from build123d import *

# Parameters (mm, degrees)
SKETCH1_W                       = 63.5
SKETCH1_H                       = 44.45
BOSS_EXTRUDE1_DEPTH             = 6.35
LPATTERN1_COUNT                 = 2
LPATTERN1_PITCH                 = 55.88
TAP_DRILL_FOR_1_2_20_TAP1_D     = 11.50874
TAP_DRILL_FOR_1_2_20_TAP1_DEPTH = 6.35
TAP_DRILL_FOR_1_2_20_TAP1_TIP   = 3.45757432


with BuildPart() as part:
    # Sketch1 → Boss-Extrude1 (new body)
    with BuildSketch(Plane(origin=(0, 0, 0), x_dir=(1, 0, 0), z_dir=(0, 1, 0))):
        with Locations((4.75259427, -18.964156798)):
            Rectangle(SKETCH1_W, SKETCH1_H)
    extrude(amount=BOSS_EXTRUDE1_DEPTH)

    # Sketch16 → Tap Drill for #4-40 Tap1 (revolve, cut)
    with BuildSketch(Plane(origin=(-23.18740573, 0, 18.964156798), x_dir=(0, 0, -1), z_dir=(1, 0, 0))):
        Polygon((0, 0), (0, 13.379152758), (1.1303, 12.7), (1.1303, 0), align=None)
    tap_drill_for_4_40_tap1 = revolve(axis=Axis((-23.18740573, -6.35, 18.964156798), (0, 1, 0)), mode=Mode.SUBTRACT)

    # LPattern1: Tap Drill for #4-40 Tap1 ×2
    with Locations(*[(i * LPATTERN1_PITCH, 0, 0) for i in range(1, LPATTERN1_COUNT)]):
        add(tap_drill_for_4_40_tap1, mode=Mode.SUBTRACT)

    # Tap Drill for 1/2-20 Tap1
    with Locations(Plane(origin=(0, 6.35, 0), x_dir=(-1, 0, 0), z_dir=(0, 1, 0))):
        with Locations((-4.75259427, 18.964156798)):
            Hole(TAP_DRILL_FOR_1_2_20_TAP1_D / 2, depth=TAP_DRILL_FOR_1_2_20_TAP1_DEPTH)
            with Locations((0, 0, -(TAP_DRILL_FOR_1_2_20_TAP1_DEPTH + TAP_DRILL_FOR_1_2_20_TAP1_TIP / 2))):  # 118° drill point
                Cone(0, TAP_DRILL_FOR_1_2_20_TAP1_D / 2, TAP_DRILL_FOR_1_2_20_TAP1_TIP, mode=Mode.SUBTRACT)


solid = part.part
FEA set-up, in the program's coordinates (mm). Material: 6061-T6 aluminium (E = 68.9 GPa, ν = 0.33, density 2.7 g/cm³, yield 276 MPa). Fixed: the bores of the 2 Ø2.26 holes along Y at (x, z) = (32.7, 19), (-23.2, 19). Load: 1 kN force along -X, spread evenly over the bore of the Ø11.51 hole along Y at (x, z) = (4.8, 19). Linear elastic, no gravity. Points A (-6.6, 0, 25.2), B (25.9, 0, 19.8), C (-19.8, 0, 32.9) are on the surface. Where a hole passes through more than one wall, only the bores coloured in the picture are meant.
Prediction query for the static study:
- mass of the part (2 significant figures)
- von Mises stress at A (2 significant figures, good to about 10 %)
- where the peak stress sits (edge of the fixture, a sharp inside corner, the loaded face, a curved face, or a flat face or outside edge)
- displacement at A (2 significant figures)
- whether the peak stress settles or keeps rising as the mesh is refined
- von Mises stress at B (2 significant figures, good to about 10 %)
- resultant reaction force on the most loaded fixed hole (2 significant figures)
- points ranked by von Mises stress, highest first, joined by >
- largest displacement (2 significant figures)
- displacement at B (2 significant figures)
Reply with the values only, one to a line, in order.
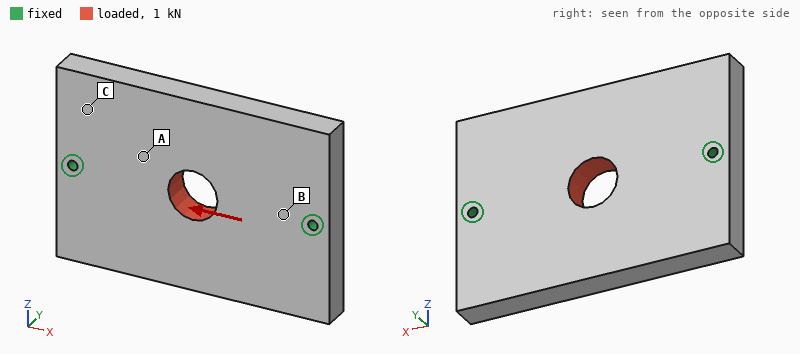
46 g
3.7 MPa
edge of the fixture
1.5 µm
keeps rising
6.7 MPa
500 N
B > A > C
2.1 µm
0.81 µm
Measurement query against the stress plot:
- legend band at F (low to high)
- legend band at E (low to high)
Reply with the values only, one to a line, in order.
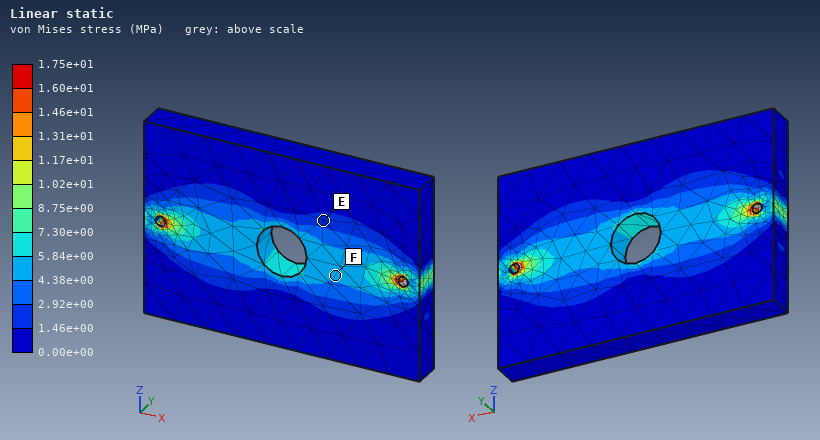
4.38e+00 to 5.84e+00 MPa
1.46e+00 to 2.92e+00 MPa
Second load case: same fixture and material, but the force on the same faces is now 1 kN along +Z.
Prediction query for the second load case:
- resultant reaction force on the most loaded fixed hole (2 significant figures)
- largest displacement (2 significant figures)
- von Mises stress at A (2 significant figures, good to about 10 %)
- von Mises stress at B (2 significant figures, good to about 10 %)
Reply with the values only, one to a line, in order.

500 N
3.8 µm
4.0 MPa
4.0 MPa
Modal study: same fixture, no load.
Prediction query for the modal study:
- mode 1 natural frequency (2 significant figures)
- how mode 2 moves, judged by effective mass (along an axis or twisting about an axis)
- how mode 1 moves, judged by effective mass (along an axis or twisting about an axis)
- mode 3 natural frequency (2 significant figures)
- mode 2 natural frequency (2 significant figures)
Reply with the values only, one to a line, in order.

4500 Hz
along Y
twisting about X
9800 Hz
5800 Hz
